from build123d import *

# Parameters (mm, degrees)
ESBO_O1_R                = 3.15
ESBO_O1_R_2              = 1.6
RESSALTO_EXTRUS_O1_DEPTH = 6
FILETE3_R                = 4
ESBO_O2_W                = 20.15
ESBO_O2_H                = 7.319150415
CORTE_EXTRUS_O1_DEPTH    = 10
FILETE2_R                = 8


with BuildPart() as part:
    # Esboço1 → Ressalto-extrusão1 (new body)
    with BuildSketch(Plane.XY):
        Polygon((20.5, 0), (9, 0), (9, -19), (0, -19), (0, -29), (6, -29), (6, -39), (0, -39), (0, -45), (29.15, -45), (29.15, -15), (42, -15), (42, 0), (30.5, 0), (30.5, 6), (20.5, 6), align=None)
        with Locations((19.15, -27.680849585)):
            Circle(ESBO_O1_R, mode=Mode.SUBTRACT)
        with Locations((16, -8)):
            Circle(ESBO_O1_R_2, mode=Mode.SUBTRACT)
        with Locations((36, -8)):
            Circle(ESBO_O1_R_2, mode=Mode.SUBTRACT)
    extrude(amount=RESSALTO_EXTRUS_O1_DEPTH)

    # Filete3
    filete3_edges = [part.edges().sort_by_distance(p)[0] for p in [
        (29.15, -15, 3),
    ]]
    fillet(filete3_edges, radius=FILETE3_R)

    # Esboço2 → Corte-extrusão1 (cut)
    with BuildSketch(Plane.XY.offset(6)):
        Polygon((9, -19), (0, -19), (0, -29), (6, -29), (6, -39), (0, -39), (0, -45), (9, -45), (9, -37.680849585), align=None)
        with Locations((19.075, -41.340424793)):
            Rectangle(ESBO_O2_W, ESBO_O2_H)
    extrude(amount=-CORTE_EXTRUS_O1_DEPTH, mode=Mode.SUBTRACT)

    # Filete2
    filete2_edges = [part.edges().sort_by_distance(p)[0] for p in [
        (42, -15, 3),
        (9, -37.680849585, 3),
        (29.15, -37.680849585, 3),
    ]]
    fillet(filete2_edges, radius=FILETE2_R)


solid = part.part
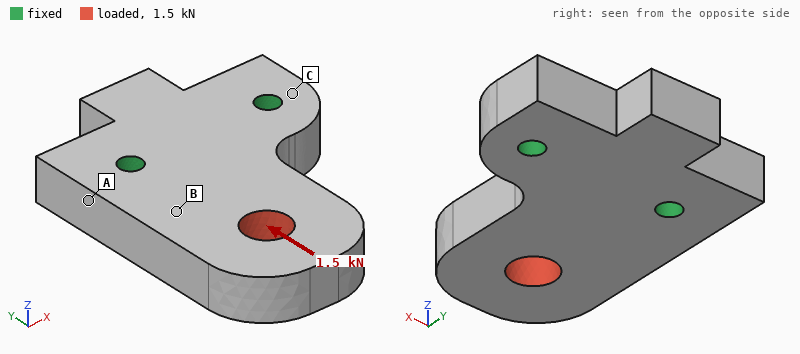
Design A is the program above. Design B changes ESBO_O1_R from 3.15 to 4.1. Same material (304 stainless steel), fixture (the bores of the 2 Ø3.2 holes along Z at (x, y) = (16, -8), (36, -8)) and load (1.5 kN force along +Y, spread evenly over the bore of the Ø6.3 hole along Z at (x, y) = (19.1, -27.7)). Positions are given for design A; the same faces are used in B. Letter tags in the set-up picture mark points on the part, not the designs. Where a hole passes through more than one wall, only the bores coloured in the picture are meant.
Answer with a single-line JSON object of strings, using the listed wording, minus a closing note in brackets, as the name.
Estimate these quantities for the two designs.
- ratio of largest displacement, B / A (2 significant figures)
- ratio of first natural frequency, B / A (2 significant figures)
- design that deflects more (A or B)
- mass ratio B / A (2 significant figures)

{"ratio of largest displacement, B / A": "1.1", "ratio of first natural frequency, B / A": "1.0", "design that deflects more": "B", "mass ratio B / A": "0.98"}
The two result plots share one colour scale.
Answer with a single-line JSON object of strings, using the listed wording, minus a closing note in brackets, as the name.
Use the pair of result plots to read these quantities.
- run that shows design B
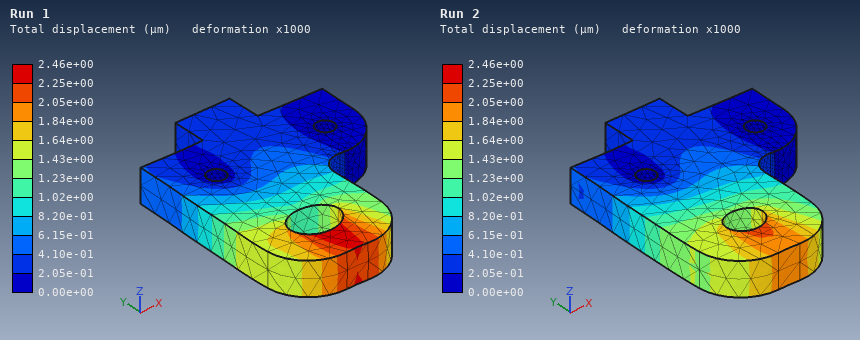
{"run that shows design B": "Run 1"}
